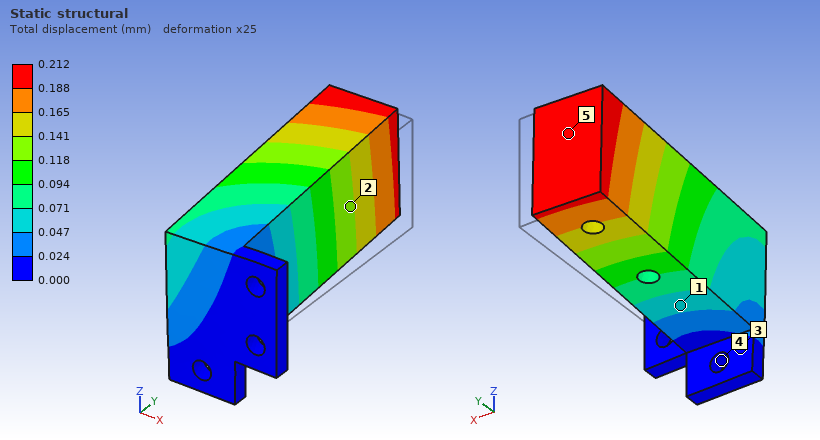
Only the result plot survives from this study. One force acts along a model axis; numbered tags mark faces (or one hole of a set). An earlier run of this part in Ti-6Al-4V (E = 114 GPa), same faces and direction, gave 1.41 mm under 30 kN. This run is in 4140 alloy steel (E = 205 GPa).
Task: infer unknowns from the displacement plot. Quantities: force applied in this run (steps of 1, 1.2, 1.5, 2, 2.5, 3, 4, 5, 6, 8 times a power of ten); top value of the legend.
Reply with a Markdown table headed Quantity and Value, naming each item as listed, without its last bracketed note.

| Quantity | Value |
|---|---|
| force applied in this run | 8 kN |
| top value of the legend | 0.212 mm |
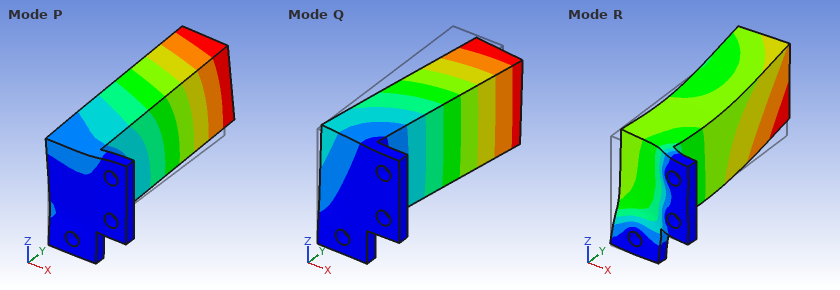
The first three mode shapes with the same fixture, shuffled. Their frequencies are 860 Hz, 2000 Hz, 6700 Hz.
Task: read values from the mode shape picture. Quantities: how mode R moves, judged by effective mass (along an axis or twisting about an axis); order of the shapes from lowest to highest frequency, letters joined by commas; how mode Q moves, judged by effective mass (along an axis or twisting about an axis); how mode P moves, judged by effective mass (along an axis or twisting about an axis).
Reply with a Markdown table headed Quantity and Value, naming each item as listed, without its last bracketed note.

| Quantity | Value |
|---|---|
| how mode R moves, judged by effective mass | along Y |
| order of the shapes from lowest to highest frequency, letters joined by commas | Q, P, R |
| how mode Q moves, judged by effective mass | along X |
| how mode P moves, judged by effective mass | along Z |
